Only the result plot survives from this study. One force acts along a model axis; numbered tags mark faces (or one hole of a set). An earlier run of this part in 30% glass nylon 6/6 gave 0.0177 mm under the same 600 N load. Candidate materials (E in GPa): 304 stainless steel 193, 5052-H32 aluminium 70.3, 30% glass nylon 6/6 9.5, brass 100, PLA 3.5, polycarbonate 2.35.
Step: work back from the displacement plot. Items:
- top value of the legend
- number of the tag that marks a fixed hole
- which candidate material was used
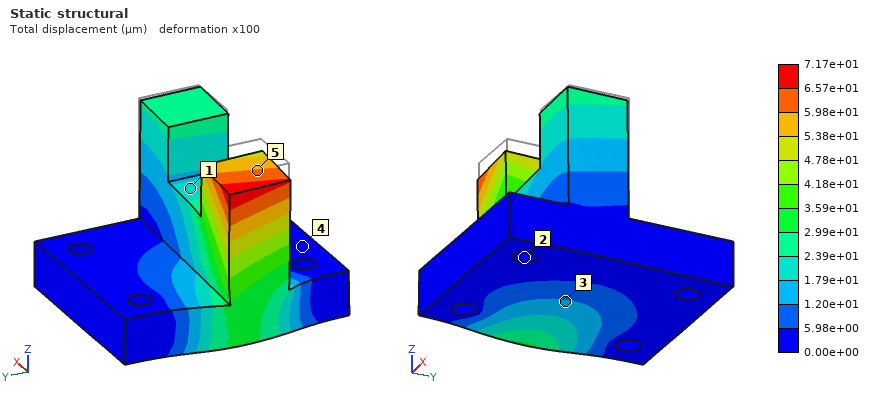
7.17e+01 µm
2
polycarbonate
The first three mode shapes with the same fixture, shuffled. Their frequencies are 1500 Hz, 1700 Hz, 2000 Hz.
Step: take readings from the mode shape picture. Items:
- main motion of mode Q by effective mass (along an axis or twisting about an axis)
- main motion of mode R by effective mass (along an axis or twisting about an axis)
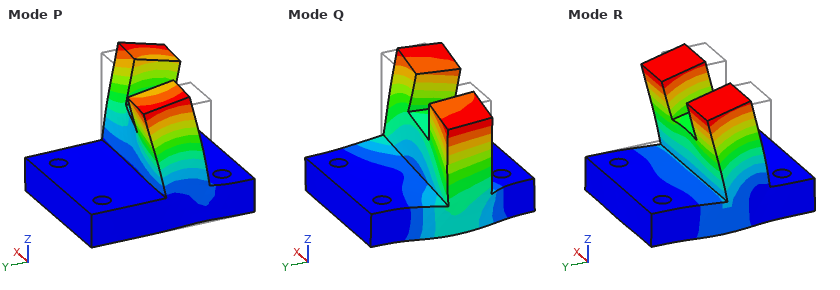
along X
along Y
